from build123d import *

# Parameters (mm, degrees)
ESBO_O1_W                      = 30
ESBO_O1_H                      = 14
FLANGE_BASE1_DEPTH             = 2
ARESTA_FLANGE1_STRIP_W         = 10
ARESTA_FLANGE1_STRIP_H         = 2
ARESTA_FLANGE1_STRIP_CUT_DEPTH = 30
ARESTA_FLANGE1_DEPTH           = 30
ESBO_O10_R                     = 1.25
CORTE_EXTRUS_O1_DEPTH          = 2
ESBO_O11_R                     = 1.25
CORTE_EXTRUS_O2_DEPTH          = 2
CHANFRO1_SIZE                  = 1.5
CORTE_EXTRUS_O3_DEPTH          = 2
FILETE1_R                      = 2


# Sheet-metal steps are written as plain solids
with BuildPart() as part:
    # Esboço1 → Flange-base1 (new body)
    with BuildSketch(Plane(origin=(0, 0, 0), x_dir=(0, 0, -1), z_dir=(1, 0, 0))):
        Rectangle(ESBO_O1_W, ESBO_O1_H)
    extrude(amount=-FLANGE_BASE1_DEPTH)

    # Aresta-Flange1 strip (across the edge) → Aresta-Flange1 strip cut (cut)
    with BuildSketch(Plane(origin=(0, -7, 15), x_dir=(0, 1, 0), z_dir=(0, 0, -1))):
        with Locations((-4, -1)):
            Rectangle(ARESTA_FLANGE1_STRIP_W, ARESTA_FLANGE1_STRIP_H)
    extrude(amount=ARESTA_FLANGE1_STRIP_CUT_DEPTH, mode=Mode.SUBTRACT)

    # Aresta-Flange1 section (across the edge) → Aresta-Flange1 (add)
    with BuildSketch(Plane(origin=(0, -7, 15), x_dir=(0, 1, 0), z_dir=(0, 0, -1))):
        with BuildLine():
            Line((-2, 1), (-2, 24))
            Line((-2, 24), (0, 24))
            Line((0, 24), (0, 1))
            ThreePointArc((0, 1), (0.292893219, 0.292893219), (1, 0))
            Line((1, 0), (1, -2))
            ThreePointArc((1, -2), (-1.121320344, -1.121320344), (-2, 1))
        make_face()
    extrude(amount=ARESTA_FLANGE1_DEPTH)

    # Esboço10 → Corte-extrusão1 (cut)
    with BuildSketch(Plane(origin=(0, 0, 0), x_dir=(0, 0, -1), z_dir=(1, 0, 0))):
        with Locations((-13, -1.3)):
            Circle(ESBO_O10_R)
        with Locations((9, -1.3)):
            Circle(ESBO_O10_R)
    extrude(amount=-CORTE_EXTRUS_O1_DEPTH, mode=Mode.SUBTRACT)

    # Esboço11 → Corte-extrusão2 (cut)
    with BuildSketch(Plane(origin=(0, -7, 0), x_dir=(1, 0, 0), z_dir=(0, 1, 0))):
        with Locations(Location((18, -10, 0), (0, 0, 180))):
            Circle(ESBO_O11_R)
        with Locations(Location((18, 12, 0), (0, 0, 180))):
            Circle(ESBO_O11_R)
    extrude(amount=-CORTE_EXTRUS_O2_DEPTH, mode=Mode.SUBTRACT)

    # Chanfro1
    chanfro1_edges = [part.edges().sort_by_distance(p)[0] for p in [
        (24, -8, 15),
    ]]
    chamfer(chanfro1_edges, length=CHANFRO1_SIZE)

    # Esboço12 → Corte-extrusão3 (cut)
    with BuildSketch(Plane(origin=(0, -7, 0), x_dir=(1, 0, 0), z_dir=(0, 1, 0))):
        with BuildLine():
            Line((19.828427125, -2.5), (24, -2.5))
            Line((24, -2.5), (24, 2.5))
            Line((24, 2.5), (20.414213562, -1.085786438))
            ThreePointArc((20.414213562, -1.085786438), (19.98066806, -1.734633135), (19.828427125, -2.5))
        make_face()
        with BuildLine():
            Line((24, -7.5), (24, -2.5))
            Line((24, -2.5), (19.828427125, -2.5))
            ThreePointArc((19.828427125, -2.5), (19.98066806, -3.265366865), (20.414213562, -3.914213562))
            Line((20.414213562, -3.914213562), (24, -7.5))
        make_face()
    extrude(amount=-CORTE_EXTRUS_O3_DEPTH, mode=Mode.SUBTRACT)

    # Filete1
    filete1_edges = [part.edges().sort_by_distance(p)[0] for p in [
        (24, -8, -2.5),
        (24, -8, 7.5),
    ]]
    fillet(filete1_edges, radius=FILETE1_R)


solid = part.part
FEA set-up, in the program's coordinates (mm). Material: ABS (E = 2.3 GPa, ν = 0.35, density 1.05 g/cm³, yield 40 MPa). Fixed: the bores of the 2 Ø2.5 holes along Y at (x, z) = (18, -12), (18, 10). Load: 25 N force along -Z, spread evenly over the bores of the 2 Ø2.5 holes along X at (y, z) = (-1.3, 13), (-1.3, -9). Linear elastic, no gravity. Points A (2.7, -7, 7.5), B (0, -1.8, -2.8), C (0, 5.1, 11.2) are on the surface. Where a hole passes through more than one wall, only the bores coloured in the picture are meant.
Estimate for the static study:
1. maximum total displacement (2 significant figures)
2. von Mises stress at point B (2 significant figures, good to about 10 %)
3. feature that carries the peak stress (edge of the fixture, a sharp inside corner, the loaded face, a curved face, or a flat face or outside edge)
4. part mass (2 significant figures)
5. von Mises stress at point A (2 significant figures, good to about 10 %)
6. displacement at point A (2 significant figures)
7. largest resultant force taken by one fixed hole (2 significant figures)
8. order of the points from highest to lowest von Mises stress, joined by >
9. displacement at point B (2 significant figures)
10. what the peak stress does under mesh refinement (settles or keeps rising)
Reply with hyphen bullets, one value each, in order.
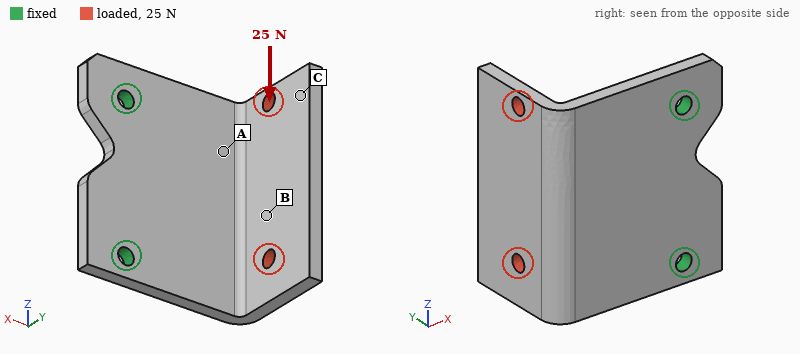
- 0.51 mm
- 2.4 MPa
- edge of the fixture
- 2.4 g
- 5.0 MPa
- 0.13 mm
- 25 N
- A > B > C
- 0.17 mm
- keeps rising
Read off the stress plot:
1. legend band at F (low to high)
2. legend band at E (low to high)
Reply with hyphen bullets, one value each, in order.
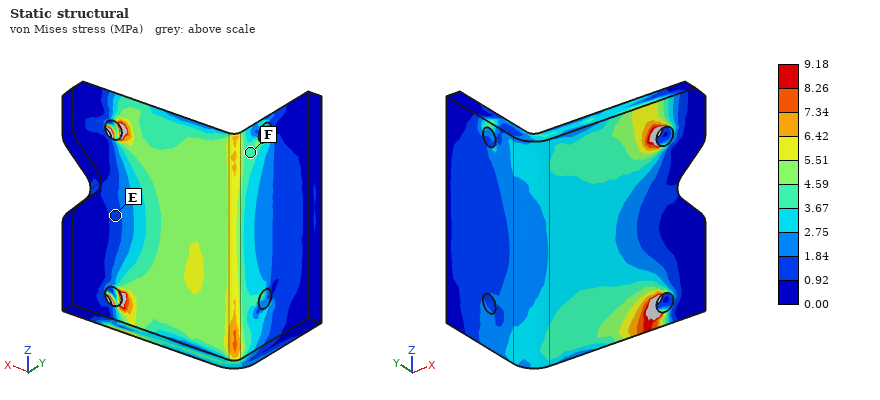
- 3.67 to 4.59 MPa
- 0.92 to 1.84 MPa
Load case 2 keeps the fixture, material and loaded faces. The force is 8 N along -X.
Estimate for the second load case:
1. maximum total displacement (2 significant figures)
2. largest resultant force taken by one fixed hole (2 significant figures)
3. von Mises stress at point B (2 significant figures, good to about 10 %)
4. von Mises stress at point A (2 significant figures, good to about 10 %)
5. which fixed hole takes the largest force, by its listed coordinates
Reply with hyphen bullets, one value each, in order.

- 0.46 mm
- 5.1 N
- 0.66 MPa
- 2.7 MPa
- (18, 10)
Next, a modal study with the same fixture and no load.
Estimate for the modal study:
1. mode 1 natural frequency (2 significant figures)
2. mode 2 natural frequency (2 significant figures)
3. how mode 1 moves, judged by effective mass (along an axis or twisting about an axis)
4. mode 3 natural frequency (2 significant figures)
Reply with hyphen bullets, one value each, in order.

- 540 Hz
- 1100 Hz
- along Y
- 1700 Hz
